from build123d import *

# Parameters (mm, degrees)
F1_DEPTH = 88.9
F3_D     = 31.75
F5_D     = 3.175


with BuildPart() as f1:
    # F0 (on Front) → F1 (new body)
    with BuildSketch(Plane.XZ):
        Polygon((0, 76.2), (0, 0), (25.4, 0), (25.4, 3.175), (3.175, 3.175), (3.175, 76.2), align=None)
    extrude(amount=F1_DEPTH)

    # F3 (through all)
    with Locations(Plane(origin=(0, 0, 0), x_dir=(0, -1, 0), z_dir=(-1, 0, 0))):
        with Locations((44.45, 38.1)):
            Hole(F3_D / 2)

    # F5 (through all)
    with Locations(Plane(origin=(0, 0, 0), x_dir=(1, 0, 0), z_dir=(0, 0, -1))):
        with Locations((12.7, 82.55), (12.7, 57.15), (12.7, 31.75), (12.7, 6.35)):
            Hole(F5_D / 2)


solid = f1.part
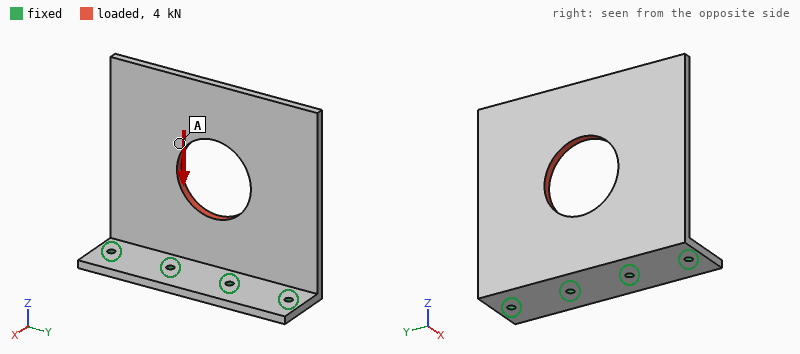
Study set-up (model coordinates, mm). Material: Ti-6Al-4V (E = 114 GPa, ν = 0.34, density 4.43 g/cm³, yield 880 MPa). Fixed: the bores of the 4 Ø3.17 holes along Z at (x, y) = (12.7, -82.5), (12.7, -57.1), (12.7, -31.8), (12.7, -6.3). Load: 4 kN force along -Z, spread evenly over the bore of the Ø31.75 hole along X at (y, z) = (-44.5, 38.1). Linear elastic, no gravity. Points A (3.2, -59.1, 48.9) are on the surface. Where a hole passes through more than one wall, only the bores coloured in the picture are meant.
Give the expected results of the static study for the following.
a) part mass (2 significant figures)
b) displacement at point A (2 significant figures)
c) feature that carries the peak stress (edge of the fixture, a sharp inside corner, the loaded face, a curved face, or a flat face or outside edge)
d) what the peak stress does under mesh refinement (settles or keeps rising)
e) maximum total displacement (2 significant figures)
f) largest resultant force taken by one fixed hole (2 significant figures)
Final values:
110 g
0.49 mm
edge of the fixture
keeps rising
0.78 mm
1.1 kN
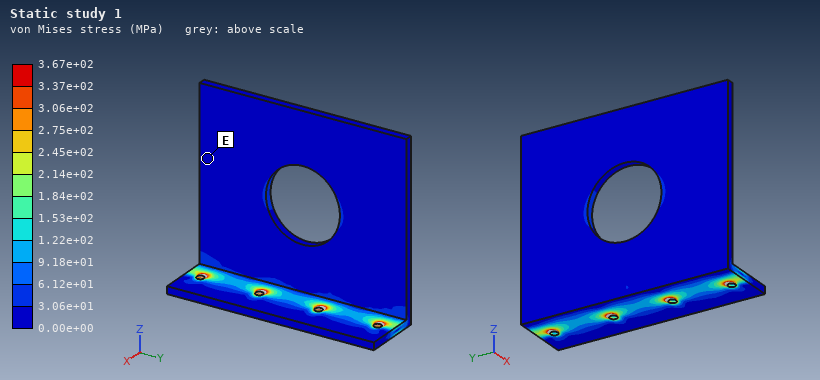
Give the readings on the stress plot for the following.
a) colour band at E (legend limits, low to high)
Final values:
0.00e+00 to 3.06e+01 MPa
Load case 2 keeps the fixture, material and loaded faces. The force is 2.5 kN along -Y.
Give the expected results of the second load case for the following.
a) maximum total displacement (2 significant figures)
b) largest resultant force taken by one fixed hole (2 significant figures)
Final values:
0.29 mm
1.2 kN
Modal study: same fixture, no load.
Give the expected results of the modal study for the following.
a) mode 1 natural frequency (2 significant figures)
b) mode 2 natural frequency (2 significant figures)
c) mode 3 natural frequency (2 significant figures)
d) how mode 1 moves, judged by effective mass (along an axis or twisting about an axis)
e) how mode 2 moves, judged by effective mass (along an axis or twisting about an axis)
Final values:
380 Hz
840 Hz
2200 Hz
along X
twisting about Z
